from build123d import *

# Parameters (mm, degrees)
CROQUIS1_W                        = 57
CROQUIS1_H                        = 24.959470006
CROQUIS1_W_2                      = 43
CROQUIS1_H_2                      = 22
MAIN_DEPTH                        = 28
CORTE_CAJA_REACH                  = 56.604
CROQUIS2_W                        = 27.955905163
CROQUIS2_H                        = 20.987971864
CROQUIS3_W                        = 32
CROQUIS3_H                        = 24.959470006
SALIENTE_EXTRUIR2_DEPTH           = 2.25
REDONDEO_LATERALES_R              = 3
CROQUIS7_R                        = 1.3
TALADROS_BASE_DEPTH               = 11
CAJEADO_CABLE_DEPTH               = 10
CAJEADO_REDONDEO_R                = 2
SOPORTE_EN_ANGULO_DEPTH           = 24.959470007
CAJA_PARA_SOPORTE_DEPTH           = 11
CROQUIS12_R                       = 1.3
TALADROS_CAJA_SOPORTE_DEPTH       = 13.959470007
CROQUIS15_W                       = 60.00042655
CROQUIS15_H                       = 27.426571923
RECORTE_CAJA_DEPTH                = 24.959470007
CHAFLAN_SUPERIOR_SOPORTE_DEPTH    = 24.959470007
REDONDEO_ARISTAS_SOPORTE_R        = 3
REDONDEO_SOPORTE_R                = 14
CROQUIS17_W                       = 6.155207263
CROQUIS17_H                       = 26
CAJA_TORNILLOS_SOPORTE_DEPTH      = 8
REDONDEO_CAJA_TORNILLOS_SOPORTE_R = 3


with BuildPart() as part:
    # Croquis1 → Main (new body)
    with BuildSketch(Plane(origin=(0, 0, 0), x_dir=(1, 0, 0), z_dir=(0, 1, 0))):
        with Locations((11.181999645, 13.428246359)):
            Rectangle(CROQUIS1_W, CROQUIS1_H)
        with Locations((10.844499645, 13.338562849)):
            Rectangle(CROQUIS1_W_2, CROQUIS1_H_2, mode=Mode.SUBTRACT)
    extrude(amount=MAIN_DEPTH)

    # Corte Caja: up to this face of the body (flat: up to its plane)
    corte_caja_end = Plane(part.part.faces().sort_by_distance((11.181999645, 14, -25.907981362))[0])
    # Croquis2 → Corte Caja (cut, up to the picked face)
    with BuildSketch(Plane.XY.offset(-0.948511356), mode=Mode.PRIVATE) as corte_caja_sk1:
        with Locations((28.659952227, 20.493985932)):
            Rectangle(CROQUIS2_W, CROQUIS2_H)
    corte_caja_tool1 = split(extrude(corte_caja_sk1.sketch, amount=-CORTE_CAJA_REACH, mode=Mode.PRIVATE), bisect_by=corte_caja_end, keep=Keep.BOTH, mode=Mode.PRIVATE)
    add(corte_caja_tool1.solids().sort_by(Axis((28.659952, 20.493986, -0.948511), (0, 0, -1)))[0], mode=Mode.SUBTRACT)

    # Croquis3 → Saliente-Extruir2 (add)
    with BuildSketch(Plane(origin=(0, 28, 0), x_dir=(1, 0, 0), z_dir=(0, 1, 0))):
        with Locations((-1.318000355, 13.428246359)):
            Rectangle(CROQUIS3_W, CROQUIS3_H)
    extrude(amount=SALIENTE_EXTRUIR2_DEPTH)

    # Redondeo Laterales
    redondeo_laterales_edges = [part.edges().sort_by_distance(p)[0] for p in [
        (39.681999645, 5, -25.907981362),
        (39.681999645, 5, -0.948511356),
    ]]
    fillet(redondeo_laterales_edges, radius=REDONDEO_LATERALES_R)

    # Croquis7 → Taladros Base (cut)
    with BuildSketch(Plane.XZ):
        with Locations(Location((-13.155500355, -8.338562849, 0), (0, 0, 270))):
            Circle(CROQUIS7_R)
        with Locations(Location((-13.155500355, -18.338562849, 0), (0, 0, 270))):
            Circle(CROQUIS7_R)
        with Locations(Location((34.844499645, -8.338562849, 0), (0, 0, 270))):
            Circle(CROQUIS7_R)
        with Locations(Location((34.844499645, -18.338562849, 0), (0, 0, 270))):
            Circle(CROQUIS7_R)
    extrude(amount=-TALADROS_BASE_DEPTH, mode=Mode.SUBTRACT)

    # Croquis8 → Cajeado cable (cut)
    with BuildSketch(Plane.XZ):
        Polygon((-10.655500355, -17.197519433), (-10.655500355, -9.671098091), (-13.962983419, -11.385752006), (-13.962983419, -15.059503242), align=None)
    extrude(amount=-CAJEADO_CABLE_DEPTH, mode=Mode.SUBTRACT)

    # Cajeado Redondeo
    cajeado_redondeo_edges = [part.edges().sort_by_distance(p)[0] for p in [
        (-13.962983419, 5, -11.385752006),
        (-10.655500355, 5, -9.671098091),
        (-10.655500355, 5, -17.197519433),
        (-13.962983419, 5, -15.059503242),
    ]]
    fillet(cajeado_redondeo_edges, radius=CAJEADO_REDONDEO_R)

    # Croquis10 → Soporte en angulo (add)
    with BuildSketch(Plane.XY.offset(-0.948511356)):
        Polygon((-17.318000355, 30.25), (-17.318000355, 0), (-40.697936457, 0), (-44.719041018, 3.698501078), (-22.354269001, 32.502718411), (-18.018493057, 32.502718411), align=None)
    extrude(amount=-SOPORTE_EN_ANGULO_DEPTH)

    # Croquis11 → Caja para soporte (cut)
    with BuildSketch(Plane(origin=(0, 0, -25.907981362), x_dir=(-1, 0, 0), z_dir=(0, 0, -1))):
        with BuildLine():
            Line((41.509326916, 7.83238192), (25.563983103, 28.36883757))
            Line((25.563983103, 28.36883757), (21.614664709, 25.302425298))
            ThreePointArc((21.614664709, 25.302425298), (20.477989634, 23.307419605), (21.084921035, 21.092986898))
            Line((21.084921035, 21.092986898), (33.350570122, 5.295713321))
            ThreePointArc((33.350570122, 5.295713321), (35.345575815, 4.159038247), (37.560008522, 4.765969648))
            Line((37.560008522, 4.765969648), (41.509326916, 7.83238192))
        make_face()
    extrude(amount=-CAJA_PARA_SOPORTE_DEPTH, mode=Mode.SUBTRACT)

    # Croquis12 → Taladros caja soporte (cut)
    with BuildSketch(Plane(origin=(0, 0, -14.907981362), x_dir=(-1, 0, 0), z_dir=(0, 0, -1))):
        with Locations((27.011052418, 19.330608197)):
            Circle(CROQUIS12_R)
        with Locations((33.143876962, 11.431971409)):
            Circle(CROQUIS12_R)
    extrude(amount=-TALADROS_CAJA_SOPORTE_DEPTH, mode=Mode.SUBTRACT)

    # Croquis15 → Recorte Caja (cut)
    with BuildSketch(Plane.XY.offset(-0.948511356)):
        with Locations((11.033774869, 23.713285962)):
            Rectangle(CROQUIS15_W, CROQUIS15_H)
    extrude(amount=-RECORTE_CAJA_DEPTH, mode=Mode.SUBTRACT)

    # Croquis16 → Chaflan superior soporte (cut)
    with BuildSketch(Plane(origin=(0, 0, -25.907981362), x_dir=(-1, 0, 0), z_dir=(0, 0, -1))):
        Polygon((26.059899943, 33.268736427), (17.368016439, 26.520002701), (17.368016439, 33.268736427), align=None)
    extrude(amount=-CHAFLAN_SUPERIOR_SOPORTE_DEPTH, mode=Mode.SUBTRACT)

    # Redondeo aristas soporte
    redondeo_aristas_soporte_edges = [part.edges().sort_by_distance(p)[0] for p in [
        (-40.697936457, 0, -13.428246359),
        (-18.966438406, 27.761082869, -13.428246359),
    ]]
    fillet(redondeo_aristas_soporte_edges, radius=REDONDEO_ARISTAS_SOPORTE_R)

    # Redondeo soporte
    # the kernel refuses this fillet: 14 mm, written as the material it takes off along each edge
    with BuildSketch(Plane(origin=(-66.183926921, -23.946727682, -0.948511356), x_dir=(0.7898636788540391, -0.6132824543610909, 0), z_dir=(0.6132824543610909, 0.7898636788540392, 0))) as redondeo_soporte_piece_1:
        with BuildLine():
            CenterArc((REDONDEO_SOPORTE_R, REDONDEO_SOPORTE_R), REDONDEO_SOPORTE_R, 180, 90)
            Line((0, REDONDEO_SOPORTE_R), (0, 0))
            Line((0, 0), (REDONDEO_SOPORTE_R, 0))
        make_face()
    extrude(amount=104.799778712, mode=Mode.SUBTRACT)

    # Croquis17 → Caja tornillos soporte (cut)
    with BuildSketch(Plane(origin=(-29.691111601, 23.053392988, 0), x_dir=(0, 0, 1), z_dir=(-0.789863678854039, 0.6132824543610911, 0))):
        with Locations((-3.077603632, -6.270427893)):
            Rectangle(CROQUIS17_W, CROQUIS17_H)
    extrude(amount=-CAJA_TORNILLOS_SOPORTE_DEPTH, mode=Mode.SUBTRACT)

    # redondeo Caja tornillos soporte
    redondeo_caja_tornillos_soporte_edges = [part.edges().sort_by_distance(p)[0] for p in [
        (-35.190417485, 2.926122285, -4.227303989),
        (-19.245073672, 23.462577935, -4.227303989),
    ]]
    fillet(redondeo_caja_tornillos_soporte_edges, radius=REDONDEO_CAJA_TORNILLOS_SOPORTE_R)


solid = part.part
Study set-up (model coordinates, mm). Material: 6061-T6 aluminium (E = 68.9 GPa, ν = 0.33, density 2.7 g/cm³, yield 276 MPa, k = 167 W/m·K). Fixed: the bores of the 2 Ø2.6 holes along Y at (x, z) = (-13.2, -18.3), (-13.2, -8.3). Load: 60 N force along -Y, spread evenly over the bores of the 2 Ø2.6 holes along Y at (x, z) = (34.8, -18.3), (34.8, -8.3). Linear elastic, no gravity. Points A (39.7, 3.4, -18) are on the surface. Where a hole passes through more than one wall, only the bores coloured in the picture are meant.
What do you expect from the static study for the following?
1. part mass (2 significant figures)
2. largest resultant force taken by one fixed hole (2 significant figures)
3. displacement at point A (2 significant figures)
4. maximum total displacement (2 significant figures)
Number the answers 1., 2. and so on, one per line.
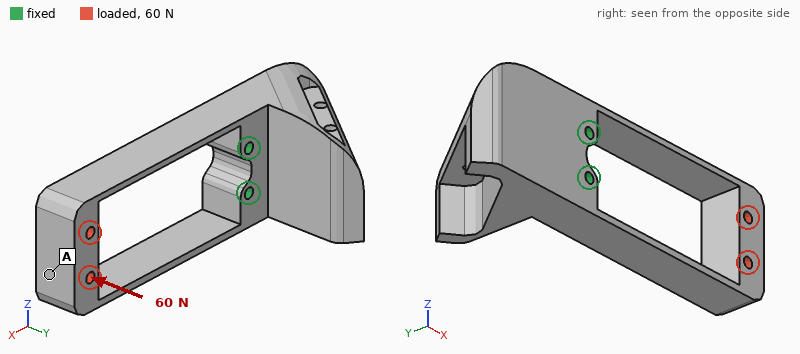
1. 35 g
2. 31 N
3. 0.17 mm
4. 0.17 mm
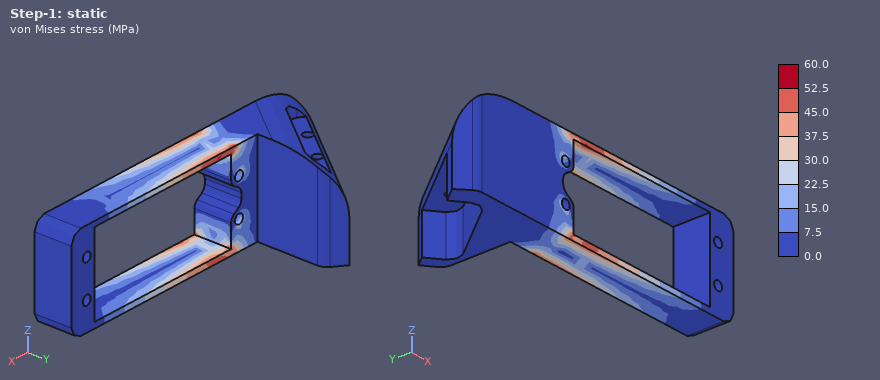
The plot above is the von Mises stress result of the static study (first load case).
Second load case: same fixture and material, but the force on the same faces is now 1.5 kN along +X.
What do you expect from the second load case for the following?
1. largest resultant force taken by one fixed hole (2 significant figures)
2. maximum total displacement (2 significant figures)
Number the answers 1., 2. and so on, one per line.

1. 820 N
2. 59 µm
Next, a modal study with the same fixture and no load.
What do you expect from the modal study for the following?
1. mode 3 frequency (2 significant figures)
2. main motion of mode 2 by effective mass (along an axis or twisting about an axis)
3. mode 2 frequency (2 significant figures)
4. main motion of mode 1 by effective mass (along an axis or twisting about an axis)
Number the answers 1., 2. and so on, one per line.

1. 3200 Hz
2. along Y
3. 1300 Hz
4. along Z
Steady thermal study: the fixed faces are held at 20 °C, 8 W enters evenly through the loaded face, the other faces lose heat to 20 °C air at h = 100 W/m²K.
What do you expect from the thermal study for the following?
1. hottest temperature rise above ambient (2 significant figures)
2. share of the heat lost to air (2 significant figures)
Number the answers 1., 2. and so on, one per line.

1. 33 K
2. 71 %
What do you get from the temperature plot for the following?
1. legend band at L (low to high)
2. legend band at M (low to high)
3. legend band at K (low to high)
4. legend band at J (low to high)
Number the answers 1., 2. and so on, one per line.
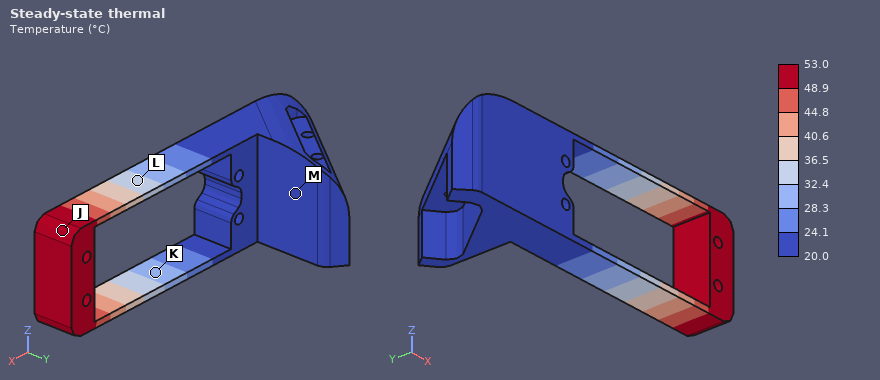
1. 32.4 to 36.5 °C
2. 20.0 to 24.1 °C
3. 28.3 to 32.4 °C
4. 48.9 to 53.0 °C
